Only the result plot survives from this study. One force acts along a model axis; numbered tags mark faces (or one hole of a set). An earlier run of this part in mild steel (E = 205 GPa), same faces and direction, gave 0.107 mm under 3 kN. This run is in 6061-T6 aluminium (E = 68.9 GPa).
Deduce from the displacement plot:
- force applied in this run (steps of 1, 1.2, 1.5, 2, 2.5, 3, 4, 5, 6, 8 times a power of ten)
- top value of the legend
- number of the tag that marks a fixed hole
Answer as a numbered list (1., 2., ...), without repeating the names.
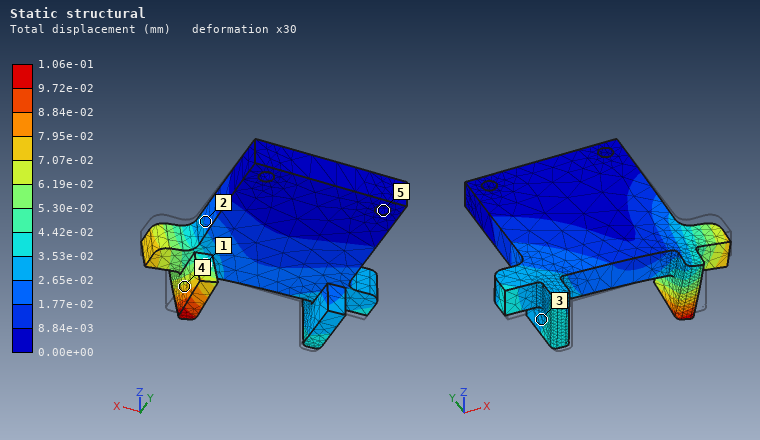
1. 1 kN
2. 1.06e-01 mm
3. 5
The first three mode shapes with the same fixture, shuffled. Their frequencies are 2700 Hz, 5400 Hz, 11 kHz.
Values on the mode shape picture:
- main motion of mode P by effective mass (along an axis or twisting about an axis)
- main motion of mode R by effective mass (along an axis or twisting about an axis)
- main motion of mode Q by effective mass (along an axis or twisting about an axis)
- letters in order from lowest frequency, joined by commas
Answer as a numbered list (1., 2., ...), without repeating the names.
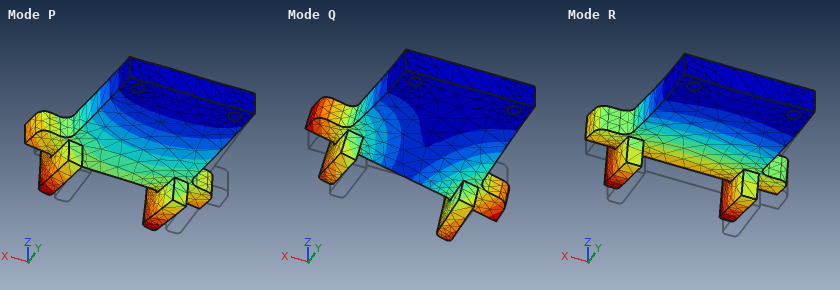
1. along X
2. along Z
3. twisting about Y
4. R, Q, P
